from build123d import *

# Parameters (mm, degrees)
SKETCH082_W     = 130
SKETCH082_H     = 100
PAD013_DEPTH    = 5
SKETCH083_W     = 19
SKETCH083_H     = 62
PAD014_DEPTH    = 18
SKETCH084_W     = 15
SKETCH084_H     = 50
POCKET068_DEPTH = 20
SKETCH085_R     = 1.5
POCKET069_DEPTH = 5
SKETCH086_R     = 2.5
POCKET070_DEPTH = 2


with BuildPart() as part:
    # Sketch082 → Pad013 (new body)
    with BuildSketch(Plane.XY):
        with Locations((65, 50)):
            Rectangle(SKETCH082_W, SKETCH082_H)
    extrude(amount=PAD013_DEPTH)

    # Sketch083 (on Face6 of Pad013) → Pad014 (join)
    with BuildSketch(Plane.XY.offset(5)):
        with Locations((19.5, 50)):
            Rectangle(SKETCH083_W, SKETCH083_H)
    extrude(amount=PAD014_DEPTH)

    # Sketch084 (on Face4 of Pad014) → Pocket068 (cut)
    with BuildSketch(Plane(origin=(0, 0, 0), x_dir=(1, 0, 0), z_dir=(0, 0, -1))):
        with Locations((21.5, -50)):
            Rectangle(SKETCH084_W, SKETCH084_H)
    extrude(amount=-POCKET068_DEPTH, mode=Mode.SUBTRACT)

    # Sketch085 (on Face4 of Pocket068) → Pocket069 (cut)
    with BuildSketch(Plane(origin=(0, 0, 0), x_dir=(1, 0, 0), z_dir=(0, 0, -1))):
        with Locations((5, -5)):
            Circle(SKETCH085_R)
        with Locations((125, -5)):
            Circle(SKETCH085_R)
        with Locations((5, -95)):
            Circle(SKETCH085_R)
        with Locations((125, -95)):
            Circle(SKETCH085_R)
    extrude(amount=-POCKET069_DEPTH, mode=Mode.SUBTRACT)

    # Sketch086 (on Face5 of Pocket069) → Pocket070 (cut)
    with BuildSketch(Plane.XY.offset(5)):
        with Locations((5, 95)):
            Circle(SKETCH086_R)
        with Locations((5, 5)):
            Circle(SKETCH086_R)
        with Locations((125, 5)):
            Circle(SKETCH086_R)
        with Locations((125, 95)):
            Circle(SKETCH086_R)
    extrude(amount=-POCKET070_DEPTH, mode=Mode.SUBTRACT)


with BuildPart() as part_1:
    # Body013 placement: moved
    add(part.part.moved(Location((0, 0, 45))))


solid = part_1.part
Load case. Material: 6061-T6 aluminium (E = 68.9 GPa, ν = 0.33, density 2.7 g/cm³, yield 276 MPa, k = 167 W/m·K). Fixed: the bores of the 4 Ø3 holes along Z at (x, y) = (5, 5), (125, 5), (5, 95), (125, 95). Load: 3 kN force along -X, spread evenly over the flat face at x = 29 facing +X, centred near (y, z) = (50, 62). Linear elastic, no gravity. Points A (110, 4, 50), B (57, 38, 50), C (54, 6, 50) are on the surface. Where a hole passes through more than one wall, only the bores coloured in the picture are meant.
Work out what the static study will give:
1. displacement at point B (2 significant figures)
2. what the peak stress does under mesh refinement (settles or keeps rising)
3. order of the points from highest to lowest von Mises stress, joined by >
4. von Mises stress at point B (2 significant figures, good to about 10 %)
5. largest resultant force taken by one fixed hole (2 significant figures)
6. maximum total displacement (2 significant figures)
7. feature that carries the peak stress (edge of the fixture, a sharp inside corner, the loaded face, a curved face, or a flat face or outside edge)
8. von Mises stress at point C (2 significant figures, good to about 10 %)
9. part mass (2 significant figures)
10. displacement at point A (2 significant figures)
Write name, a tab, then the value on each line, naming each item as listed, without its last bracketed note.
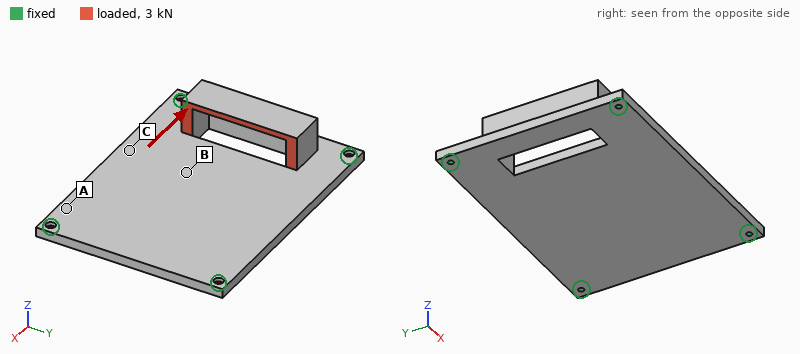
displacement at point B	0.27 mm
what the peak stress does under mesh refinement	keeps rising
order of the points from highest to lowest von Mises stress, joined by >	C > B > A
von Mises stress at point B	27 MPa
largest resultant force taken by one fixed hole	1.0 kN
maximum total displacement	0.34 mm
feature that carries the peak stress	edge of the fixture
von Mises stress at point C	45 MPa
part mass	190 g
displacement at point A	0.052 mm
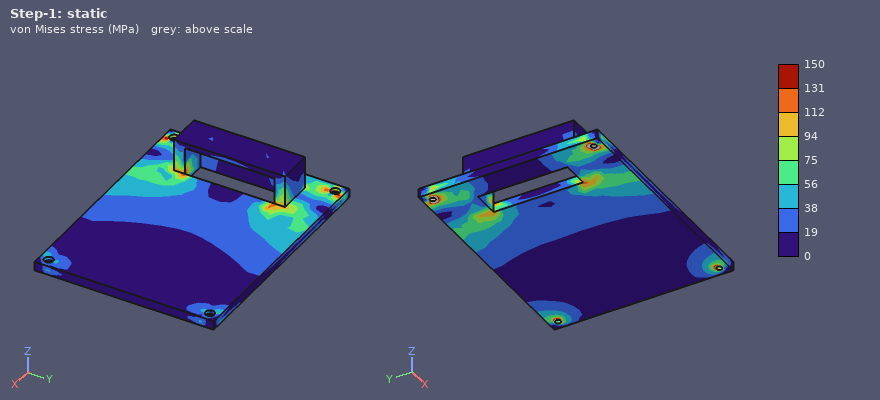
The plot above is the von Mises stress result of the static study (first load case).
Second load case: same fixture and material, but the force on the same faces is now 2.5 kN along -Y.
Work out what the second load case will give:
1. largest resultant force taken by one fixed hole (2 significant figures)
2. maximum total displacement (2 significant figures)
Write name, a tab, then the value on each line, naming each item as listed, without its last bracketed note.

largest resultant force taken by one fixed hole	1.2 kN
maximum total displacement	62 µm
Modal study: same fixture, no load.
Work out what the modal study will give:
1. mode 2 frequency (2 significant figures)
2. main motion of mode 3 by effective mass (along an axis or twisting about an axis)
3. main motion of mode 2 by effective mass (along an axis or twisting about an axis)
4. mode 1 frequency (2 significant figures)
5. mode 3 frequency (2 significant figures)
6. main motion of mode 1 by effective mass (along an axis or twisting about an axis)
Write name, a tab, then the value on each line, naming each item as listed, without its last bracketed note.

mode 2 frequency	2000 Hz
main motion of mode 3 by effective mass	twisting about Y
main motion of mode 2 by effective mass	twisting about X
mode 1 frequency	1100 Hz
mode 3 frequency	2500 Hz
main motion of mode 1 by effective mass	along Z
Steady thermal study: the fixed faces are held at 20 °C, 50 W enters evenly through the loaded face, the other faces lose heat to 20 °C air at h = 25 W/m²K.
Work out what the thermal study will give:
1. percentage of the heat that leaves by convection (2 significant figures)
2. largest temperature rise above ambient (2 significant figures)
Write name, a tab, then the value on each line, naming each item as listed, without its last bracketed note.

percentage of the heat that leaves by convection	21 %
largest temperature rise above ambient	41 K
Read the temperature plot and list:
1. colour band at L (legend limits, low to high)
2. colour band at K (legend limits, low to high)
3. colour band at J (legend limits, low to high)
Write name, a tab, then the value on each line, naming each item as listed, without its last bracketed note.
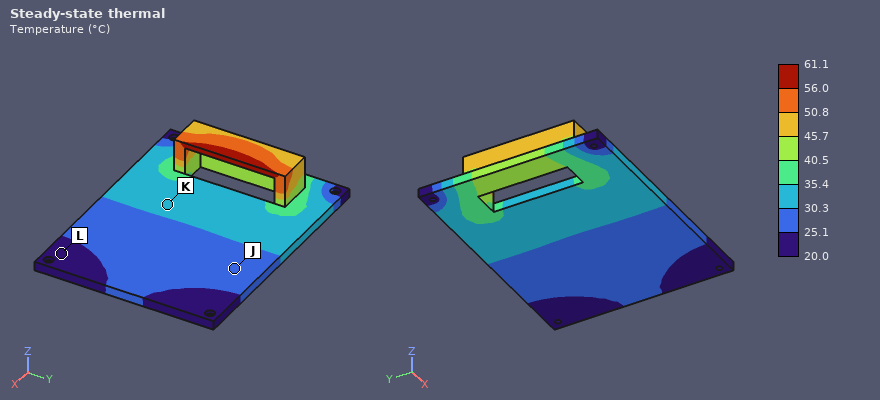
colour band at L	20.0 to 25.1 °C
colour band at K	30.3 to 35.4 °C
colour band at J	25.1 to 30.3 °C
